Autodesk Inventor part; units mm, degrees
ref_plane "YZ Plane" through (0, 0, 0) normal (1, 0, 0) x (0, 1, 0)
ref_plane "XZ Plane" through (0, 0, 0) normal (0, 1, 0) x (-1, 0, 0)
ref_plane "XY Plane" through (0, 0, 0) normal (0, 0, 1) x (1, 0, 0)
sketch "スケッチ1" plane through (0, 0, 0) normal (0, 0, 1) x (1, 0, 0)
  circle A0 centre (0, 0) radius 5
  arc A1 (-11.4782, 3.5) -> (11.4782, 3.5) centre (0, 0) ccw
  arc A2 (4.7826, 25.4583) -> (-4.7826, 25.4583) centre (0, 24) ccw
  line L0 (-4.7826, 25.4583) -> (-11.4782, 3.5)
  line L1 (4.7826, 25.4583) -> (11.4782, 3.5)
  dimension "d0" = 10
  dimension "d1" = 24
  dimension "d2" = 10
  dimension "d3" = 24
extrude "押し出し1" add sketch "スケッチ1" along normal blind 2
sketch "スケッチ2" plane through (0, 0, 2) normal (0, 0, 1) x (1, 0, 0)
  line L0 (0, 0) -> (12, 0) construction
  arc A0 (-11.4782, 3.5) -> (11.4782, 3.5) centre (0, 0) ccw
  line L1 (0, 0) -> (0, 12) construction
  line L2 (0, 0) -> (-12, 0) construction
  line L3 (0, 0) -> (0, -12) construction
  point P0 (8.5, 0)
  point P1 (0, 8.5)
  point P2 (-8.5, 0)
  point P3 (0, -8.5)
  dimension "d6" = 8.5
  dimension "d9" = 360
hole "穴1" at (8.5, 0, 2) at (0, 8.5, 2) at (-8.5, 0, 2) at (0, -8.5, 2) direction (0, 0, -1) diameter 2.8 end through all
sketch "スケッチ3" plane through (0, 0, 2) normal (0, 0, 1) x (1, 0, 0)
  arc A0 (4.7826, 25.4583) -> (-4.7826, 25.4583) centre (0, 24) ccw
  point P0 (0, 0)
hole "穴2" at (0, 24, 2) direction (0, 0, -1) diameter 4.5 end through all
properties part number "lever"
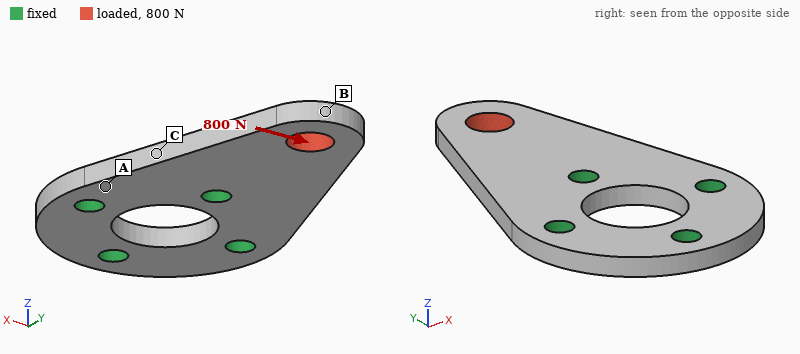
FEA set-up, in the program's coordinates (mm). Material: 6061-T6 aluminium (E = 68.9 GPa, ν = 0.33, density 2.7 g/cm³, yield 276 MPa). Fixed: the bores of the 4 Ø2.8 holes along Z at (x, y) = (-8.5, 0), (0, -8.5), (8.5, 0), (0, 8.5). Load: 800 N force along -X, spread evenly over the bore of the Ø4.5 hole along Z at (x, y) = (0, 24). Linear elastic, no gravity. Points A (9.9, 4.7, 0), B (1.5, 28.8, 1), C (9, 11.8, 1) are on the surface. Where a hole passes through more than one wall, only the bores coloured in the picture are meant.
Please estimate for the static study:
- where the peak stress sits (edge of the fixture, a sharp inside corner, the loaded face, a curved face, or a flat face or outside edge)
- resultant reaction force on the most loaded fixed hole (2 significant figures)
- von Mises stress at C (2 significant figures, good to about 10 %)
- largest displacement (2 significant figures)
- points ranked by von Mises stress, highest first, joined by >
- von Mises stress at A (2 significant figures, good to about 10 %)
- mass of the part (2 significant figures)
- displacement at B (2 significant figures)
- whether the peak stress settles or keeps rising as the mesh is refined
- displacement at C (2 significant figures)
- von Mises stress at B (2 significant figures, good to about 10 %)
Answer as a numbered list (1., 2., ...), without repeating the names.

1. edge of the fixture
2. 730 N
3. 110 MPa
4. 69 µm
5. C > A > B
6. 65 MPa
7. 3.1 g
8. 69 µm
9. keeps rising
10. 14 µm
11. 28 MPa
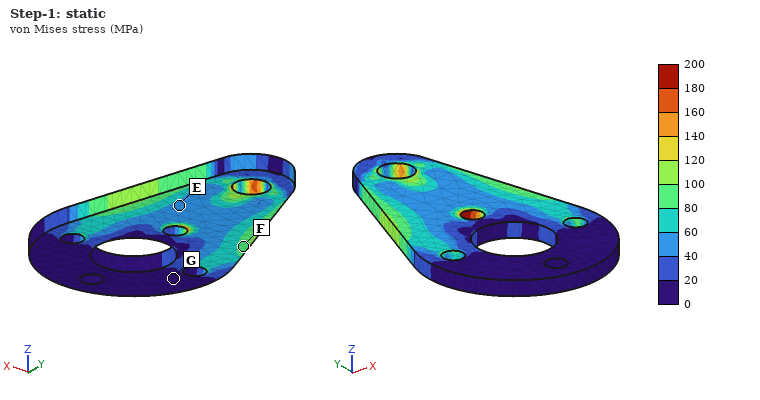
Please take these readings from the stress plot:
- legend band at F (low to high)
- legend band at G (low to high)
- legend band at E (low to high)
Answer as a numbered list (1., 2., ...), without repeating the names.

1. 80 to 100 MPa
2. 0 to 20 MPa
3. 40 to 60 MPa
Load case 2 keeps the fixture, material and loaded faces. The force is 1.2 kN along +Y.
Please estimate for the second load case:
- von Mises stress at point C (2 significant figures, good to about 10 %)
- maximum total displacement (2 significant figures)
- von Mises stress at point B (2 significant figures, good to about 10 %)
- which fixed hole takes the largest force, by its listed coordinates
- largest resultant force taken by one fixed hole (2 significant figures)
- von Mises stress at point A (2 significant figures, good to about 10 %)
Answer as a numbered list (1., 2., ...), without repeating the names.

1. 22 MPa
2. 17 µm
3. 54 MPa
4. (0, 8.5)
5. 760 N
6. 18 MPa
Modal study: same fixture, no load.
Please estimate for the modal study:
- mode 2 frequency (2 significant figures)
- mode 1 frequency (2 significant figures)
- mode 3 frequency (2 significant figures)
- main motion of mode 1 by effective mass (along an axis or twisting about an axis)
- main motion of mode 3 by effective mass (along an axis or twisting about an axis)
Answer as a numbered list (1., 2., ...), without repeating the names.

1. 15 kHz
2. 5800 Hz
3. 23 kHz
4. along Z
5. along Z
